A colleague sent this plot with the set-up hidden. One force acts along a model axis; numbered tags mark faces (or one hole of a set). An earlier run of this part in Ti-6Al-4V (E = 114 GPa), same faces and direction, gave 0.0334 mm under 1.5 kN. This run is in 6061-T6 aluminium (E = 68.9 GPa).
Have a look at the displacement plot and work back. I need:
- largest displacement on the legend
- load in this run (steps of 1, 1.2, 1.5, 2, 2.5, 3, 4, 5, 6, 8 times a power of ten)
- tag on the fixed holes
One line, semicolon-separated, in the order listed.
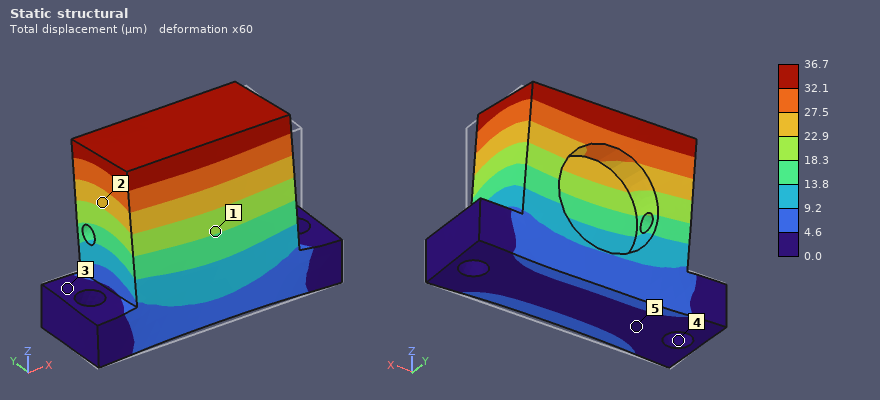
36.7 µm; 1 kN; 4
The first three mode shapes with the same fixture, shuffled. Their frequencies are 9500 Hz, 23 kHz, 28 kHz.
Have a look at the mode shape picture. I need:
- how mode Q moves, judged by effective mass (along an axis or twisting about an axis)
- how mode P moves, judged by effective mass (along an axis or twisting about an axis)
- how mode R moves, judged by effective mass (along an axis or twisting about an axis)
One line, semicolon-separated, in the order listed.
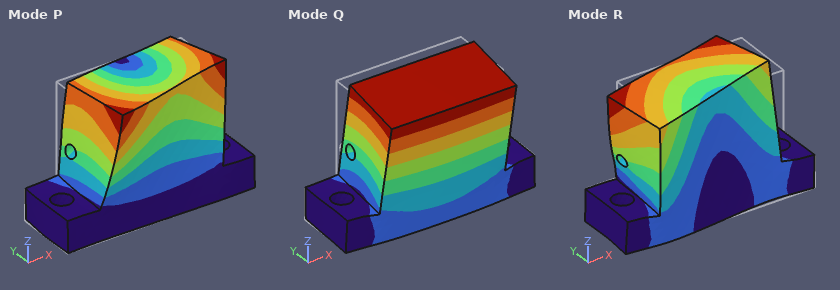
along Y; along X; along X
